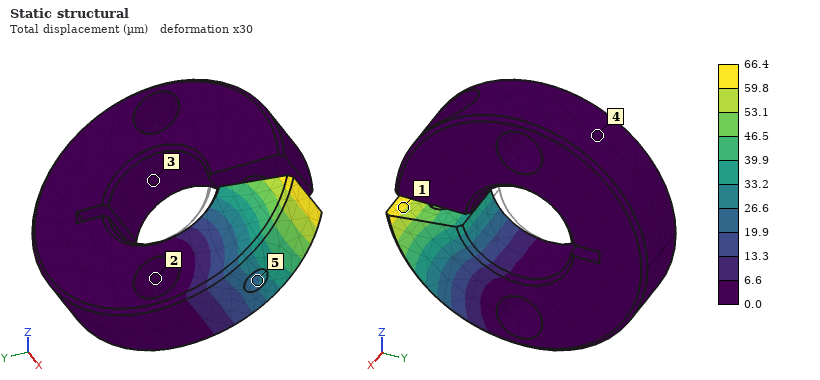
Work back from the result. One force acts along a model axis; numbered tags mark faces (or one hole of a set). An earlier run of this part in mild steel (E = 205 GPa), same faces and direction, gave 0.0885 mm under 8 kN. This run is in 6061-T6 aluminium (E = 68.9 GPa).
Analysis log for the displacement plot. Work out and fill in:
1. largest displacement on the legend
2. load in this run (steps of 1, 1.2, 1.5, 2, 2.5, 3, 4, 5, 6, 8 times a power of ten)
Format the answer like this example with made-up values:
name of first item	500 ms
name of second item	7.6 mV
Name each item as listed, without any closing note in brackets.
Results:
largest displacement on the legend	66.4 µm
load in this run	2 kN
